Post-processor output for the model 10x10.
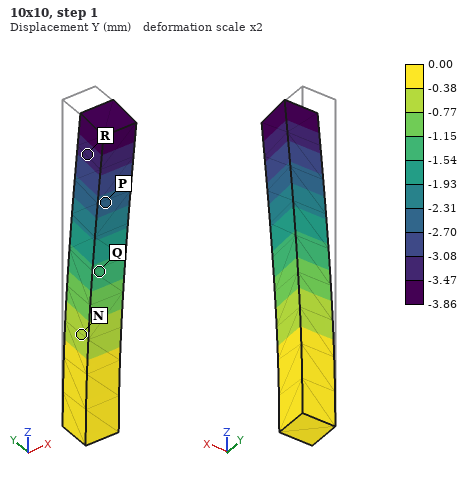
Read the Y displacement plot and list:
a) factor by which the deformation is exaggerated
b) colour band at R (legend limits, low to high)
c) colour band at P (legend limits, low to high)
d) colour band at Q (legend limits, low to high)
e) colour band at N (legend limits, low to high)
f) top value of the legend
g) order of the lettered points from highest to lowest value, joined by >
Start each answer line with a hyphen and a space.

- 2
- -3.47 to -3.08 mm
- -2.70 to -2.31 mm
- -1.54 to -1.15 mm
- -0.77 to -0.38 mm
- 0.00 mm
- N > Q > P > R
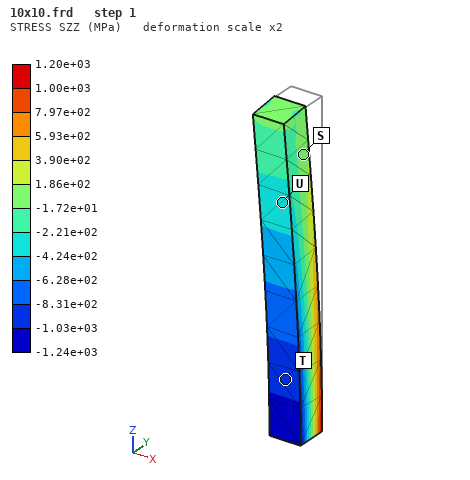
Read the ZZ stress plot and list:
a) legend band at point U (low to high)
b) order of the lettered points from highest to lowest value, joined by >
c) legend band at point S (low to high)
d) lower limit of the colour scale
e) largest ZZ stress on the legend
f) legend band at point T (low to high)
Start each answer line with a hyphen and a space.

- -4.24e+02 to -2.21e+02 MPa
- S > U > T
- -1.72e+01 to 1.86e+02 MPa
- -1.24e+03 MPa
- 1.20e+03 MPa
- -1.03e+03 to -8.31e+02 MPa
